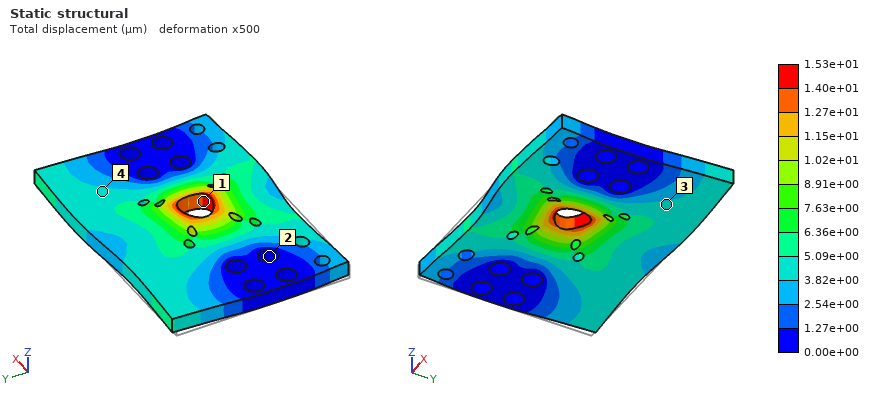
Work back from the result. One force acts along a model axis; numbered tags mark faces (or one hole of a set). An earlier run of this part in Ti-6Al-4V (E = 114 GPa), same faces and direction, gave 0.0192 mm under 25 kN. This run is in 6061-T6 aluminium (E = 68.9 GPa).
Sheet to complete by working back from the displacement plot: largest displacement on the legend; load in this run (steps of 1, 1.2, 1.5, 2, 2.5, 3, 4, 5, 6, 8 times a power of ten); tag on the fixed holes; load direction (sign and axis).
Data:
1.53e+01 µm
12 kN
2
+X
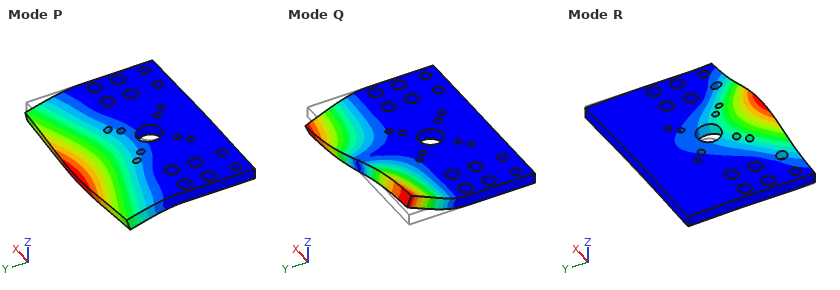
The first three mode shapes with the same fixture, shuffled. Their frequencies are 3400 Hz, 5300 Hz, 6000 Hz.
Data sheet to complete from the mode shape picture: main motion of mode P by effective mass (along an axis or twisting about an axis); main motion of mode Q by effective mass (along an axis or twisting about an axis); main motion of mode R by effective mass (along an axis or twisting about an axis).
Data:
along Z
twisting about Y
along Z
